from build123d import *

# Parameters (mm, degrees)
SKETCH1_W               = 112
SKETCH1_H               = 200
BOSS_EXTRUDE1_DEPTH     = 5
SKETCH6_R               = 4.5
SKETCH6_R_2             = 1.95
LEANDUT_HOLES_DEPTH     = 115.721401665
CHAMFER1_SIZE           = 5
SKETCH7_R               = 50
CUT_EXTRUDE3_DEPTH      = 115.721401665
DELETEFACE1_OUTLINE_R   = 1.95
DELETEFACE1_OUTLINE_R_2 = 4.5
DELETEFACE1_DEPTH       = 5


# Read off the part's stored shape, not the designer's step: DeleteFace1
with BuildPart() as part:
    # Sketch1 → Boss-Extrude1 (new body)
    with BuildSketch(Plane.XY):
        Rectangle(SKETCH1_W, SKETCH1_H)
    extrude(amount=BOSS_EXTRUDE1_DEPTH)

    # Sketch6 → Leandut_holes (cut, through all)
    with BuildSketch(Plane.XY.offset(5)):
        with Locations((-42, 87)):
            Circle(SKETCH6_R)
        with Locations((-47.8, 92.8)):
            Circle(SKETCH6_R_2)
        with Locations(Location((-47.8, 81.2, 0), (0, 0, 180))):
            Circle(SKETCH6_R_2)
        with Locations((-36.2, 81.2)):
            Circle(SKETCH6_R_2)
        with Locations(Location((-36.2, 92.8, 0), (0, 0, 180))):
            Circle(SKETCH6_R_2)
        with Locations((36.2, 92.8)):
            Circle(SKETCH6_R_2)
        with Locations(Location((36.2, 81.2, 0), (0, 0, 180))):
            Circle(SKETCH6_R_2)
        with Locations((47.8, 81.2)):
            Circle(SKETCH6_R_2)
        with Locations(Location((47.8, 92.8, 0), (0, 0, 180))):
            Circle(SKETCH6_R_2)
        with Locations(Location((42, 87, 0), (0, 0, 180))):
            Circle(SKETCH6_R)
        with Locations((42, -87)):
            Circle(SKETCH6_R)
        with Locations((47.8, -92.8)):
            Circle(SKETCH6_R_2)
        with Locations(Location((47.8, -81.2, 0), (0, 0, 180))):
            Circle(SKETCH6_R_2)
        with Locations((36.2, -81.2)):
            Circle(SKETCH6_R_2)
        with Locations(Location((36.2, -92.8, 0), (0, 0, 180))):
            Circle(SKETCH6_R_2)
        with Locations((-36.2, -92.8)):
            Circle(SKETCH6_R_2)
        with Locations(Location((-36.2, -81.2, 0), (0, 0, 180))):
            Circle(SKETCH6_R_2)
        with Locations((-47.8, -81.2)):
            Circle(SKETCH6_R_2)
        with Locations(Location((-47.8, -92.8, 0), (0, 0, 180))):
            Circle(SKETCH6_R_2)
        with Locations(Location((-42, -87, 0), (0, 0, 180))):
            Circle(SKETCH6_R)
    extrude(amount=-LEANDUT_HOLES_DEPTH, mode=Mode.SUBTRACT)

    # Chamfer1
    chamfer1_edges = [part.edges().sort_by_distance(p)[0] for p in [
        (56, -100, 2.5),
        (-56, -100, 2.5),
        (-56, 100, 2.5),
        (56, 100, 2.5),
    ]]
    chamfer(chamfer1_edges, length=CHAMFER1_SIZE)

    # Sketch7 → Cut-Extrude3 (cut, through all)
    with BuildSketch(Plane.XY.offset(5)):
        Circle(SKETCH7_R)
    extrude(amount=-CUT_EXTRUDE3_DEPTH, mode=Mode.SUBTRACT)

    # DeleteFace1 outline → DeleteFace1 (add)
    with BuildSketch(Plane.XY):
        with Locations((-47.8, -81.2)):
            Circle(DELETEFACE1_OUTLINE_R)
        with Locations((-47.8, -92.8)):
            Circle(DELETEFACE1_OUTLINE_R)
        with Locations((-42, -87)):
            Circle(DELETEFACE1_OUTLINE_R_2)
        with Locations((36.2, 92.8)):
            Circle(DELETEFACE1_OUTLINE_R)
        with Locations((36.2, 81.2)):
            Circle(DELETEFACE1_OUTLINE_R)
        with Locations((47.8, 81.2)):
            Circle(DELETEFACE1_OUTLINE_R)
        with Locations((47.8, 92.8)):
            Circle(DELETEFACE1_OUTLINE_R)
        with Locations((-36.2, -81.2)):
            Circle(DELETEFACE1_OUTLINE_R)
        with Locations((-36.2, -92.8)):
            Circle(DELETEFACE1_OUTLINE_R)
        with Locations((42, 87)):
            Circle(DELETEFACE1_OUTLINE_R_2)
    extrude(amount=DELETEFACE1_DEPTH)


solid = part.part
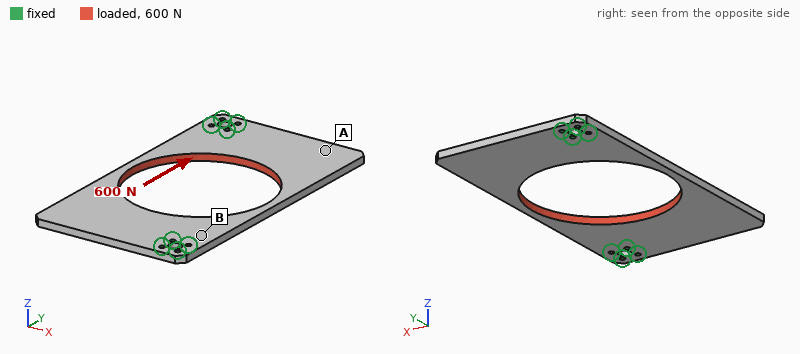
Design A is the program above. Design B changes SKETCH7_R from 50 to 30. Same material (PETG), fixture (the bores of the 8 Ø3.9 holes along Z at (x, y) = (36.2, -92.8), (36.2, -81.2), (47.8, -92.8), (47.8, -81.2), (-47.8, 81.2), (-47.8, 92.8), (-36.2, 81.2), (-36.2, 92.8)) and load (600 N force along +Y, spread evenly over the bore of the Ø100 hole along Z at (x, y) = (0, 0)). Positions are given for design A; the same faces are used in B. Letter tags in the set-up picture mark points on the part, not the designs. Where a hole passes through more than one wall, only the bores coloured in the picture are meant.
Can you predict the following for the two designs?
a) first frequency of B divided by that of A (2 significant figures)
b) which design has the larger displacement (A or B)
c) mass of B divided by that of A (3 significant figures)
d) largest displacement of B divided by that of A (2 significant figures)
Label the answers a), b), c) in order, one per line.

a) 0.99
b) A
c) 1.35
d) 0.52
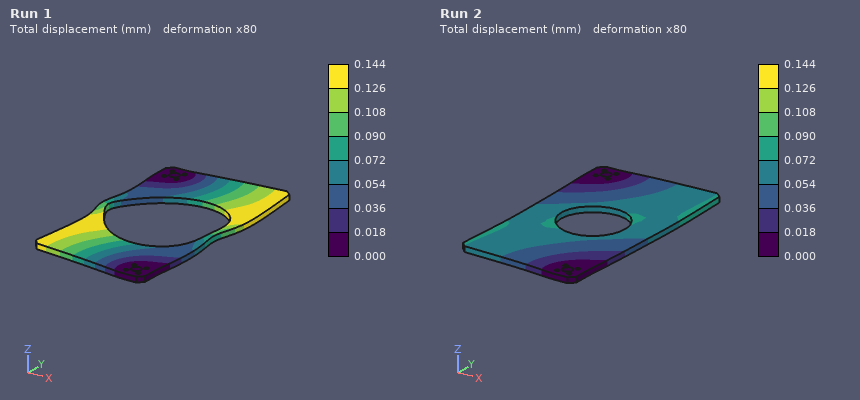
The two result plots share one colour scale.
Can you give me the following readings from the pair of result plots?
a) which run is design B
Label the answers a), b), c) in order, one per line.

a) Run 2
